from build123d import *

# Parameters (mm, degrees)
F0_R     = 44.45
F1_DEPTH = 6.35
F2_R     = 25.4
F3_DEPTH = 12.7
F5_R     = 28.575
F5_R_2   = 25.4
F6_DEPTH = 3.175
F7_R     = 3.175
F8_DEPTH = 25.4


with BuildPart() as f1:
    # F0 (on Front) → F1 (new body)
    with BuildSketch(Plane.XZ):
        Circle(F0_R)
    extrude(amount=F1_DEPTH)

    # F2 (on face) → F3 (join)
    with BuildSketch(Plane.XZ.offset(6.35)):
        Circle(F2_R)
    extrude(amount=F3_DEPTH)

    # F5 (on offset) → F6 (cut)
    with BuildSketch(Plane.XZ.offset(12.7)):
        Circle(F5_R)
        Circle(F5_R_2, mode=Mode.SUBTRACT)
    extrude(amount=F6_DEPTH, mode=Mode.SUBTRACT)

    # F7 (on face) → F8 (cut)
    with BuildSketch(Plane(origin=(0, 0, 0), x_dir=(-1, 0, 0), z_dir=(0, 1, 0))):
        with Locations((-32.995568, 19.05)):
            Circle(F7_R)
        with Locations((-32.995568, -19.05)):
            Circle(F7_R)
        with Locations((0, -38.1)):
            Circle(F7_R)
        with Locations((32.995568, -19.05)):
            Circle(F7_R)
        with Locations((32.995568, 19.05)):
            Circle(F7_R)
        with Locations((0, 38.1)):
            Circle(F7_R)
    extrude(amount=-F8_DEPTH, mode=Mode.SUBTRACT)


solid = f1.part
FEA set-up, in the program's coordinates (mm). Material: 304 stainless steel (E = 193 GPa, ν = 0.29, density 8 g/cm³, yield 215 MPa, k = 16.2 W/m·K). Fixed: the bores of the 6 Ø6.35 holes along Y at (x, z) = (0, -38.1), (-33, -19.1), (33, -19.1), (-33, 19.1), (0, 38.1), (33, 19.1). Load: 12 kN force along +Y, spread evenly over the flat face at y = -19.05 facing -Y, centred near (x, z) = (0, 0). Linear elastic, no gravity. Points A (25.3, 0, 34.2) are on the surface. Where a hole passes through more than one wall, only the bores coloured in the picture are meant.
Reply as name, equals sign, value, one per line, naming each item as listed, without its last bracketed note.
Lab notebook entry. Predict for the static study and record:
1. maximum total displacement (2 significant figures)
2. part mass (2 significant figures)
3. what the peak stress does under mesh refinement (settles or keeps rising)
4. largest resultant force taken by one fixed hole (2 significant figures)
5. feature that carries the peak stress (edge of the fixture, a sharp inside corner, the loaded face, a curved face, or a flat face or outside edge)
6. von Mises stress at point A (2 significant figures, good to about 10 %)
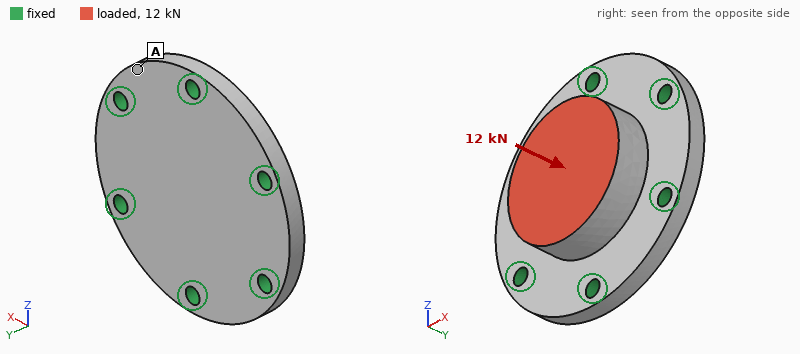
maximum total displacement = 11 µm
part mass = 510 g
what the peak stress does under mesh refinement = keeps rising
largest resultant force taken by one fixed hole = 2.2 kN
feature that carries the peak stress = edge of the fixture
von Mises stress at point A = 13 MPa
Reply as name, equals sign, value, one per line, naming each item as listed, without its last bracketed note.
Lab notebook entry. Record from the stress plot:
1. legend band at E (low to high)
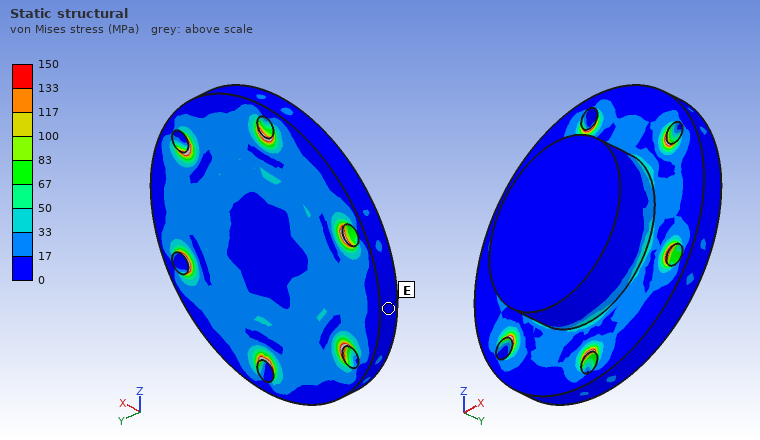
legend band at E = 0 to 17 MPa
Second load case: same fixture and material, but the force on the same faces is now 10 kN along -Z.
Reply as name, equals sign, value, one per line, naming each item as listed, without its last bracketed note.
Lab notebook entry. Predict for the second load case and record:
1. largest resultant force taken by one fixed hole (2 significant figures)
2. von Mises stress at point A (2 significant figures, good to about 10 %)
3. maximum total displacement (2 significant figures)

largest resultant force taken by one fixed hole = 2.9 kN
von Mises stress at point A = 15 MPa
maximum total displacement = 8.5 µm
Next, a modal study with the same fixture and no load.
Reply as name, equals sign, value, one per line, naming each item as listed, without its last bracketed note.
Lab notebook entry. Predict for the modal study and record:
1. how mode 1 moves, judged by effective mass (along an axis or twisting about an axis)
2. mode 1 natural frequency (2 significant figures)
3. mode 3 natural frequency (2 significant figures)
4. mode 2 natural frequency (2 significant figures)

how mode 1 moves, judged by effective mass = along Y
mode 1 natural frequency = 9500 Hz
mode 3 natural frequency = 14 kHz
mode 2 natural frequency = 14 kHz
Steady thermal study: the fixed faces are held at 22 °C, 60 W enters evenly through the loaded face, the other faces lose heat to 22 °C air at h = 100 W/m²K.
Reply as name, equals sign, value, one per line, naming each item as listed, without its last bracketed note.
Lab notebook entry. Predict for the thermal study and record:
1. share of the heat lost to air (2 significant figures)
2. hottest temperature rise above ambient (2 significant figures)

share of the heat lost to air = 48 %
hottest temperature rise above ambient = 68 K
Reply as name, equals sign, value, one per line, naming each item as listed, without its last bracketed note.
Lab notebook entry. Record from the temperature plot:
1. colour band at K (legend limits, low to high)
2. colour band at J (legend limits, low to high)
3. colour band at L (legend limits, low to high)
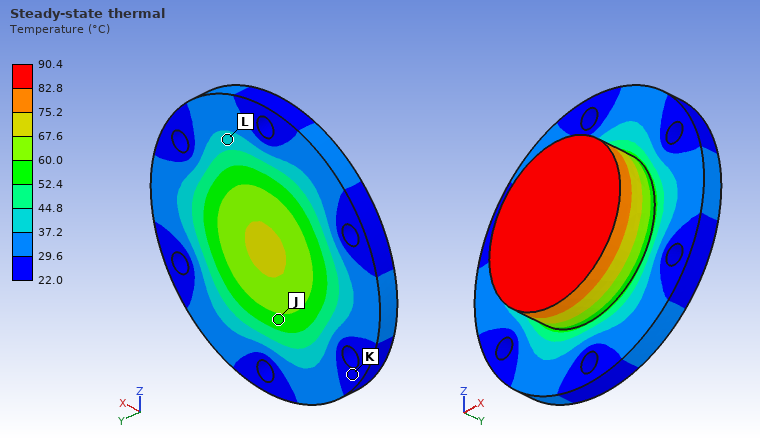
colour band at K = 22.0 to 29.6 °C
colour band at J = 52.4 to 60.0 °C
colour band at L = 37.2 to 44.8 °C
